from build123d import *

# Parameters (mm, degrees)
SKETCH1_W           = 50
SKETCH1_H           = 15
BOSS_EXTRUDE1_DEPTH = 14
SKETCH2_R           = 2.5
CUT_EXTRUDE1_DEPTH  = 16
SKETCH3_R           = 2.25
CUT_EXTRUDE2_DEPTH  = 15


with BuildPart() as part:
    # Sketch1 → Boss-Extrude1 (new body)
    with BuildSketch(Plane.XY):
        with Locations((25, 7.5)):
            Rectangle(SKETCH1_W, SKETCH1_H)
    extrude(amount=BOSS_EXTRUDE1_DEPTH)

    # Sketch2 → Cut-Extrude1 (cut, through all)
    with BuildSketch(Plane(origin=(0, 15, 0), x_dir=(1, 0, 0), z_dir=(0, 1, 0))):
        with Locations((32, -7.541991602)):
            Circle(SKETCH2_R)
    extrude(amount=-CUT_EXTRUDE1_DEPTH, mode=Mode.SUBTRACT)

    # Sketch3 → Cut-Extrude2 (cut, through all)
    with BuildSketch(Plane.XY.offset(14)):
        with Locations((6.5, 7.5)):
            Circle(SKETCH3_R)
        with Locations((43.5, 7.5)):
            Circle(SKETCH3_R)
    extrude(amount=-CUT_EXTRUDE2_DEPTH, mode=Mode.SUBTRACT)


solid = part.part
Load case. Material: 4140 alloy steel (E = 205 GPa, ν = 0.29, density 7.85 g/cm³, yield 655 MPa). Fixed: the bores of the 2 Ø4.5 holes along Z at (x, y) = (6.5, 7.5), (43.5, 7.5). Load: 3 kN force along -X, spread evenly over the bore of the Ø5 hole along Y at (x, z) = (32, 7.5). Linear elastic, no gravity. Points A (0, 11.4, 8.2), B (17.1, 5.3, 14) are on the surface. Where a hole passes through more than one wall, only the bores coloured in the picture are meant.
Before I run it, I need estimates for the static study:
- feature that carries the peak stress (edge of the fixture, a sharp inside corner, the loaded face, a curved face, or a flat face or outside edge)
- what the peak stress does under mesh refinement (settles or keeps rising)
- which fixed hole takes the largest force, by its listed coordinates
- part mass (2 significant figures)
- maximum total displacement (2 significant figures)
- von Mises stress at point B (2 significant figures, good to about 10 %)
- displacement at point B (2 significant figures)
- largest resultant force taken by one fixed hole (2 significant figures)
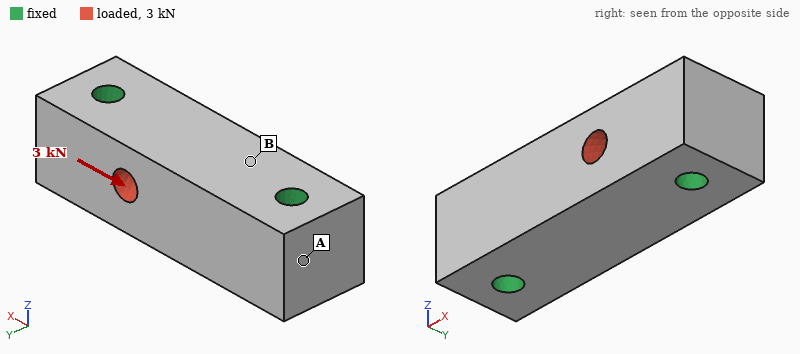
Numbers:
edge of the fixture
keeps rising
(43.5, 7.5)
77 g
0.77 µm
5.8 MPa
0.29 µm
2.0 kN
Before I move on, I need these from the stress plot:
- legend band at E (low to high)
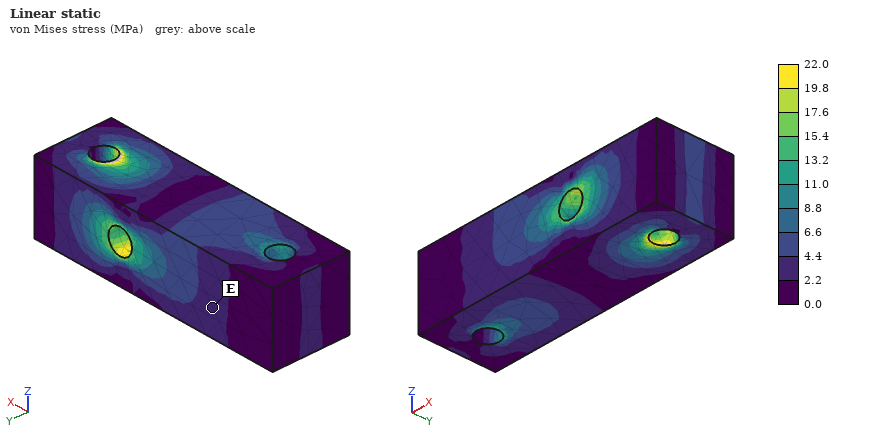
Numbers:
2.2 to 4.4 MPa
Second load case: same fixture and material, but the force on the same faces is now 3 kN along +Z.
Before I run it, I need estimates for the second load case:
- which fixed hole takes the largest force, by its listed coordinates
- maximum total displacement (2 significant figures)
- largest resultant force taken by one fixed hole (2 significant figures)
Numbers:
(43.5, 7.5)
2.8 µm
2.2 kN
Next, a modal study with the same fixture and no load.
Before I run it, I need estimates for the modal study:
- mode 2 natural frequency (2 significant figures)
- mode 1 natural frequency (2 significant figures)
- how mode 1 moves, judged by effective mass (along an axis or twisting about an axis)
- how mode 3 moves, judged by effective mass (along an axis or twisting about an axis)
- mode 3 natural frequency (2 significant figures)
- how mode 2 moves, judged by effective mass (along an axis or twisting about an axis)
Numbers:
31 kHz
28 kHz
along Y
twisting about X
39 kHz
along Z
